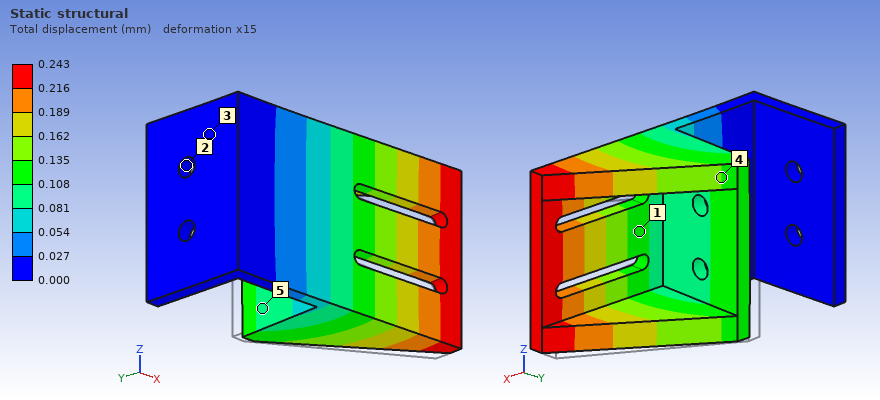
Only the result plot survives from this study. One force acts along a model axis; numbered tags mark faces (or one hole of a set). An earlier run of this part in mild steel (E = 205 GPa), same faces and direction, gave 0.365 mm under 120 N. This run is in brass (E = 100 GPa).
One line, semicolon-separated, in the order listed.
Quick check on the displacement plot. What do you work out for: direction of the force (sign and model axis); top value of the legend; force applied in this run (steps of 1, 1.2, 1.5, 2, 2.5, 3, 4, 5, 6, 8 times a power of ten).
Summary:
-Y; 0.243 mm; 40 N
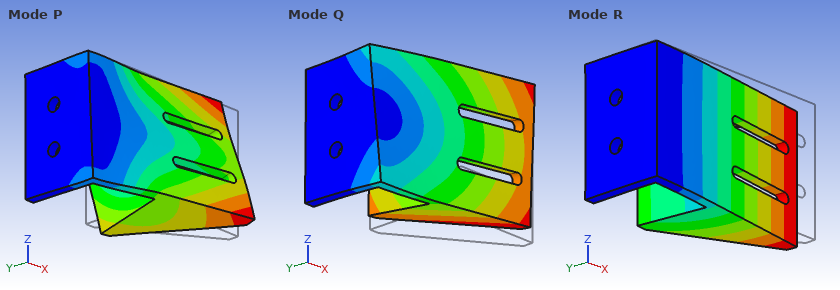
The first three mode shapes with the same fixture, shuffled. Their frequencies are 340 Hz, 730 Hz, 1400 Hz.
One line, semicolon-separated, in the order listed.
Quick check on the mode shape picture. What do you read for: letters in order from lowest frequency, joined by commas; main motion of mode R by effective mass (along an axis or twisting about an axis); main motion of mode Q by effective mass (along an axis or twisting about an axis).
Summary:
R, Q, P; along Y; along Z
